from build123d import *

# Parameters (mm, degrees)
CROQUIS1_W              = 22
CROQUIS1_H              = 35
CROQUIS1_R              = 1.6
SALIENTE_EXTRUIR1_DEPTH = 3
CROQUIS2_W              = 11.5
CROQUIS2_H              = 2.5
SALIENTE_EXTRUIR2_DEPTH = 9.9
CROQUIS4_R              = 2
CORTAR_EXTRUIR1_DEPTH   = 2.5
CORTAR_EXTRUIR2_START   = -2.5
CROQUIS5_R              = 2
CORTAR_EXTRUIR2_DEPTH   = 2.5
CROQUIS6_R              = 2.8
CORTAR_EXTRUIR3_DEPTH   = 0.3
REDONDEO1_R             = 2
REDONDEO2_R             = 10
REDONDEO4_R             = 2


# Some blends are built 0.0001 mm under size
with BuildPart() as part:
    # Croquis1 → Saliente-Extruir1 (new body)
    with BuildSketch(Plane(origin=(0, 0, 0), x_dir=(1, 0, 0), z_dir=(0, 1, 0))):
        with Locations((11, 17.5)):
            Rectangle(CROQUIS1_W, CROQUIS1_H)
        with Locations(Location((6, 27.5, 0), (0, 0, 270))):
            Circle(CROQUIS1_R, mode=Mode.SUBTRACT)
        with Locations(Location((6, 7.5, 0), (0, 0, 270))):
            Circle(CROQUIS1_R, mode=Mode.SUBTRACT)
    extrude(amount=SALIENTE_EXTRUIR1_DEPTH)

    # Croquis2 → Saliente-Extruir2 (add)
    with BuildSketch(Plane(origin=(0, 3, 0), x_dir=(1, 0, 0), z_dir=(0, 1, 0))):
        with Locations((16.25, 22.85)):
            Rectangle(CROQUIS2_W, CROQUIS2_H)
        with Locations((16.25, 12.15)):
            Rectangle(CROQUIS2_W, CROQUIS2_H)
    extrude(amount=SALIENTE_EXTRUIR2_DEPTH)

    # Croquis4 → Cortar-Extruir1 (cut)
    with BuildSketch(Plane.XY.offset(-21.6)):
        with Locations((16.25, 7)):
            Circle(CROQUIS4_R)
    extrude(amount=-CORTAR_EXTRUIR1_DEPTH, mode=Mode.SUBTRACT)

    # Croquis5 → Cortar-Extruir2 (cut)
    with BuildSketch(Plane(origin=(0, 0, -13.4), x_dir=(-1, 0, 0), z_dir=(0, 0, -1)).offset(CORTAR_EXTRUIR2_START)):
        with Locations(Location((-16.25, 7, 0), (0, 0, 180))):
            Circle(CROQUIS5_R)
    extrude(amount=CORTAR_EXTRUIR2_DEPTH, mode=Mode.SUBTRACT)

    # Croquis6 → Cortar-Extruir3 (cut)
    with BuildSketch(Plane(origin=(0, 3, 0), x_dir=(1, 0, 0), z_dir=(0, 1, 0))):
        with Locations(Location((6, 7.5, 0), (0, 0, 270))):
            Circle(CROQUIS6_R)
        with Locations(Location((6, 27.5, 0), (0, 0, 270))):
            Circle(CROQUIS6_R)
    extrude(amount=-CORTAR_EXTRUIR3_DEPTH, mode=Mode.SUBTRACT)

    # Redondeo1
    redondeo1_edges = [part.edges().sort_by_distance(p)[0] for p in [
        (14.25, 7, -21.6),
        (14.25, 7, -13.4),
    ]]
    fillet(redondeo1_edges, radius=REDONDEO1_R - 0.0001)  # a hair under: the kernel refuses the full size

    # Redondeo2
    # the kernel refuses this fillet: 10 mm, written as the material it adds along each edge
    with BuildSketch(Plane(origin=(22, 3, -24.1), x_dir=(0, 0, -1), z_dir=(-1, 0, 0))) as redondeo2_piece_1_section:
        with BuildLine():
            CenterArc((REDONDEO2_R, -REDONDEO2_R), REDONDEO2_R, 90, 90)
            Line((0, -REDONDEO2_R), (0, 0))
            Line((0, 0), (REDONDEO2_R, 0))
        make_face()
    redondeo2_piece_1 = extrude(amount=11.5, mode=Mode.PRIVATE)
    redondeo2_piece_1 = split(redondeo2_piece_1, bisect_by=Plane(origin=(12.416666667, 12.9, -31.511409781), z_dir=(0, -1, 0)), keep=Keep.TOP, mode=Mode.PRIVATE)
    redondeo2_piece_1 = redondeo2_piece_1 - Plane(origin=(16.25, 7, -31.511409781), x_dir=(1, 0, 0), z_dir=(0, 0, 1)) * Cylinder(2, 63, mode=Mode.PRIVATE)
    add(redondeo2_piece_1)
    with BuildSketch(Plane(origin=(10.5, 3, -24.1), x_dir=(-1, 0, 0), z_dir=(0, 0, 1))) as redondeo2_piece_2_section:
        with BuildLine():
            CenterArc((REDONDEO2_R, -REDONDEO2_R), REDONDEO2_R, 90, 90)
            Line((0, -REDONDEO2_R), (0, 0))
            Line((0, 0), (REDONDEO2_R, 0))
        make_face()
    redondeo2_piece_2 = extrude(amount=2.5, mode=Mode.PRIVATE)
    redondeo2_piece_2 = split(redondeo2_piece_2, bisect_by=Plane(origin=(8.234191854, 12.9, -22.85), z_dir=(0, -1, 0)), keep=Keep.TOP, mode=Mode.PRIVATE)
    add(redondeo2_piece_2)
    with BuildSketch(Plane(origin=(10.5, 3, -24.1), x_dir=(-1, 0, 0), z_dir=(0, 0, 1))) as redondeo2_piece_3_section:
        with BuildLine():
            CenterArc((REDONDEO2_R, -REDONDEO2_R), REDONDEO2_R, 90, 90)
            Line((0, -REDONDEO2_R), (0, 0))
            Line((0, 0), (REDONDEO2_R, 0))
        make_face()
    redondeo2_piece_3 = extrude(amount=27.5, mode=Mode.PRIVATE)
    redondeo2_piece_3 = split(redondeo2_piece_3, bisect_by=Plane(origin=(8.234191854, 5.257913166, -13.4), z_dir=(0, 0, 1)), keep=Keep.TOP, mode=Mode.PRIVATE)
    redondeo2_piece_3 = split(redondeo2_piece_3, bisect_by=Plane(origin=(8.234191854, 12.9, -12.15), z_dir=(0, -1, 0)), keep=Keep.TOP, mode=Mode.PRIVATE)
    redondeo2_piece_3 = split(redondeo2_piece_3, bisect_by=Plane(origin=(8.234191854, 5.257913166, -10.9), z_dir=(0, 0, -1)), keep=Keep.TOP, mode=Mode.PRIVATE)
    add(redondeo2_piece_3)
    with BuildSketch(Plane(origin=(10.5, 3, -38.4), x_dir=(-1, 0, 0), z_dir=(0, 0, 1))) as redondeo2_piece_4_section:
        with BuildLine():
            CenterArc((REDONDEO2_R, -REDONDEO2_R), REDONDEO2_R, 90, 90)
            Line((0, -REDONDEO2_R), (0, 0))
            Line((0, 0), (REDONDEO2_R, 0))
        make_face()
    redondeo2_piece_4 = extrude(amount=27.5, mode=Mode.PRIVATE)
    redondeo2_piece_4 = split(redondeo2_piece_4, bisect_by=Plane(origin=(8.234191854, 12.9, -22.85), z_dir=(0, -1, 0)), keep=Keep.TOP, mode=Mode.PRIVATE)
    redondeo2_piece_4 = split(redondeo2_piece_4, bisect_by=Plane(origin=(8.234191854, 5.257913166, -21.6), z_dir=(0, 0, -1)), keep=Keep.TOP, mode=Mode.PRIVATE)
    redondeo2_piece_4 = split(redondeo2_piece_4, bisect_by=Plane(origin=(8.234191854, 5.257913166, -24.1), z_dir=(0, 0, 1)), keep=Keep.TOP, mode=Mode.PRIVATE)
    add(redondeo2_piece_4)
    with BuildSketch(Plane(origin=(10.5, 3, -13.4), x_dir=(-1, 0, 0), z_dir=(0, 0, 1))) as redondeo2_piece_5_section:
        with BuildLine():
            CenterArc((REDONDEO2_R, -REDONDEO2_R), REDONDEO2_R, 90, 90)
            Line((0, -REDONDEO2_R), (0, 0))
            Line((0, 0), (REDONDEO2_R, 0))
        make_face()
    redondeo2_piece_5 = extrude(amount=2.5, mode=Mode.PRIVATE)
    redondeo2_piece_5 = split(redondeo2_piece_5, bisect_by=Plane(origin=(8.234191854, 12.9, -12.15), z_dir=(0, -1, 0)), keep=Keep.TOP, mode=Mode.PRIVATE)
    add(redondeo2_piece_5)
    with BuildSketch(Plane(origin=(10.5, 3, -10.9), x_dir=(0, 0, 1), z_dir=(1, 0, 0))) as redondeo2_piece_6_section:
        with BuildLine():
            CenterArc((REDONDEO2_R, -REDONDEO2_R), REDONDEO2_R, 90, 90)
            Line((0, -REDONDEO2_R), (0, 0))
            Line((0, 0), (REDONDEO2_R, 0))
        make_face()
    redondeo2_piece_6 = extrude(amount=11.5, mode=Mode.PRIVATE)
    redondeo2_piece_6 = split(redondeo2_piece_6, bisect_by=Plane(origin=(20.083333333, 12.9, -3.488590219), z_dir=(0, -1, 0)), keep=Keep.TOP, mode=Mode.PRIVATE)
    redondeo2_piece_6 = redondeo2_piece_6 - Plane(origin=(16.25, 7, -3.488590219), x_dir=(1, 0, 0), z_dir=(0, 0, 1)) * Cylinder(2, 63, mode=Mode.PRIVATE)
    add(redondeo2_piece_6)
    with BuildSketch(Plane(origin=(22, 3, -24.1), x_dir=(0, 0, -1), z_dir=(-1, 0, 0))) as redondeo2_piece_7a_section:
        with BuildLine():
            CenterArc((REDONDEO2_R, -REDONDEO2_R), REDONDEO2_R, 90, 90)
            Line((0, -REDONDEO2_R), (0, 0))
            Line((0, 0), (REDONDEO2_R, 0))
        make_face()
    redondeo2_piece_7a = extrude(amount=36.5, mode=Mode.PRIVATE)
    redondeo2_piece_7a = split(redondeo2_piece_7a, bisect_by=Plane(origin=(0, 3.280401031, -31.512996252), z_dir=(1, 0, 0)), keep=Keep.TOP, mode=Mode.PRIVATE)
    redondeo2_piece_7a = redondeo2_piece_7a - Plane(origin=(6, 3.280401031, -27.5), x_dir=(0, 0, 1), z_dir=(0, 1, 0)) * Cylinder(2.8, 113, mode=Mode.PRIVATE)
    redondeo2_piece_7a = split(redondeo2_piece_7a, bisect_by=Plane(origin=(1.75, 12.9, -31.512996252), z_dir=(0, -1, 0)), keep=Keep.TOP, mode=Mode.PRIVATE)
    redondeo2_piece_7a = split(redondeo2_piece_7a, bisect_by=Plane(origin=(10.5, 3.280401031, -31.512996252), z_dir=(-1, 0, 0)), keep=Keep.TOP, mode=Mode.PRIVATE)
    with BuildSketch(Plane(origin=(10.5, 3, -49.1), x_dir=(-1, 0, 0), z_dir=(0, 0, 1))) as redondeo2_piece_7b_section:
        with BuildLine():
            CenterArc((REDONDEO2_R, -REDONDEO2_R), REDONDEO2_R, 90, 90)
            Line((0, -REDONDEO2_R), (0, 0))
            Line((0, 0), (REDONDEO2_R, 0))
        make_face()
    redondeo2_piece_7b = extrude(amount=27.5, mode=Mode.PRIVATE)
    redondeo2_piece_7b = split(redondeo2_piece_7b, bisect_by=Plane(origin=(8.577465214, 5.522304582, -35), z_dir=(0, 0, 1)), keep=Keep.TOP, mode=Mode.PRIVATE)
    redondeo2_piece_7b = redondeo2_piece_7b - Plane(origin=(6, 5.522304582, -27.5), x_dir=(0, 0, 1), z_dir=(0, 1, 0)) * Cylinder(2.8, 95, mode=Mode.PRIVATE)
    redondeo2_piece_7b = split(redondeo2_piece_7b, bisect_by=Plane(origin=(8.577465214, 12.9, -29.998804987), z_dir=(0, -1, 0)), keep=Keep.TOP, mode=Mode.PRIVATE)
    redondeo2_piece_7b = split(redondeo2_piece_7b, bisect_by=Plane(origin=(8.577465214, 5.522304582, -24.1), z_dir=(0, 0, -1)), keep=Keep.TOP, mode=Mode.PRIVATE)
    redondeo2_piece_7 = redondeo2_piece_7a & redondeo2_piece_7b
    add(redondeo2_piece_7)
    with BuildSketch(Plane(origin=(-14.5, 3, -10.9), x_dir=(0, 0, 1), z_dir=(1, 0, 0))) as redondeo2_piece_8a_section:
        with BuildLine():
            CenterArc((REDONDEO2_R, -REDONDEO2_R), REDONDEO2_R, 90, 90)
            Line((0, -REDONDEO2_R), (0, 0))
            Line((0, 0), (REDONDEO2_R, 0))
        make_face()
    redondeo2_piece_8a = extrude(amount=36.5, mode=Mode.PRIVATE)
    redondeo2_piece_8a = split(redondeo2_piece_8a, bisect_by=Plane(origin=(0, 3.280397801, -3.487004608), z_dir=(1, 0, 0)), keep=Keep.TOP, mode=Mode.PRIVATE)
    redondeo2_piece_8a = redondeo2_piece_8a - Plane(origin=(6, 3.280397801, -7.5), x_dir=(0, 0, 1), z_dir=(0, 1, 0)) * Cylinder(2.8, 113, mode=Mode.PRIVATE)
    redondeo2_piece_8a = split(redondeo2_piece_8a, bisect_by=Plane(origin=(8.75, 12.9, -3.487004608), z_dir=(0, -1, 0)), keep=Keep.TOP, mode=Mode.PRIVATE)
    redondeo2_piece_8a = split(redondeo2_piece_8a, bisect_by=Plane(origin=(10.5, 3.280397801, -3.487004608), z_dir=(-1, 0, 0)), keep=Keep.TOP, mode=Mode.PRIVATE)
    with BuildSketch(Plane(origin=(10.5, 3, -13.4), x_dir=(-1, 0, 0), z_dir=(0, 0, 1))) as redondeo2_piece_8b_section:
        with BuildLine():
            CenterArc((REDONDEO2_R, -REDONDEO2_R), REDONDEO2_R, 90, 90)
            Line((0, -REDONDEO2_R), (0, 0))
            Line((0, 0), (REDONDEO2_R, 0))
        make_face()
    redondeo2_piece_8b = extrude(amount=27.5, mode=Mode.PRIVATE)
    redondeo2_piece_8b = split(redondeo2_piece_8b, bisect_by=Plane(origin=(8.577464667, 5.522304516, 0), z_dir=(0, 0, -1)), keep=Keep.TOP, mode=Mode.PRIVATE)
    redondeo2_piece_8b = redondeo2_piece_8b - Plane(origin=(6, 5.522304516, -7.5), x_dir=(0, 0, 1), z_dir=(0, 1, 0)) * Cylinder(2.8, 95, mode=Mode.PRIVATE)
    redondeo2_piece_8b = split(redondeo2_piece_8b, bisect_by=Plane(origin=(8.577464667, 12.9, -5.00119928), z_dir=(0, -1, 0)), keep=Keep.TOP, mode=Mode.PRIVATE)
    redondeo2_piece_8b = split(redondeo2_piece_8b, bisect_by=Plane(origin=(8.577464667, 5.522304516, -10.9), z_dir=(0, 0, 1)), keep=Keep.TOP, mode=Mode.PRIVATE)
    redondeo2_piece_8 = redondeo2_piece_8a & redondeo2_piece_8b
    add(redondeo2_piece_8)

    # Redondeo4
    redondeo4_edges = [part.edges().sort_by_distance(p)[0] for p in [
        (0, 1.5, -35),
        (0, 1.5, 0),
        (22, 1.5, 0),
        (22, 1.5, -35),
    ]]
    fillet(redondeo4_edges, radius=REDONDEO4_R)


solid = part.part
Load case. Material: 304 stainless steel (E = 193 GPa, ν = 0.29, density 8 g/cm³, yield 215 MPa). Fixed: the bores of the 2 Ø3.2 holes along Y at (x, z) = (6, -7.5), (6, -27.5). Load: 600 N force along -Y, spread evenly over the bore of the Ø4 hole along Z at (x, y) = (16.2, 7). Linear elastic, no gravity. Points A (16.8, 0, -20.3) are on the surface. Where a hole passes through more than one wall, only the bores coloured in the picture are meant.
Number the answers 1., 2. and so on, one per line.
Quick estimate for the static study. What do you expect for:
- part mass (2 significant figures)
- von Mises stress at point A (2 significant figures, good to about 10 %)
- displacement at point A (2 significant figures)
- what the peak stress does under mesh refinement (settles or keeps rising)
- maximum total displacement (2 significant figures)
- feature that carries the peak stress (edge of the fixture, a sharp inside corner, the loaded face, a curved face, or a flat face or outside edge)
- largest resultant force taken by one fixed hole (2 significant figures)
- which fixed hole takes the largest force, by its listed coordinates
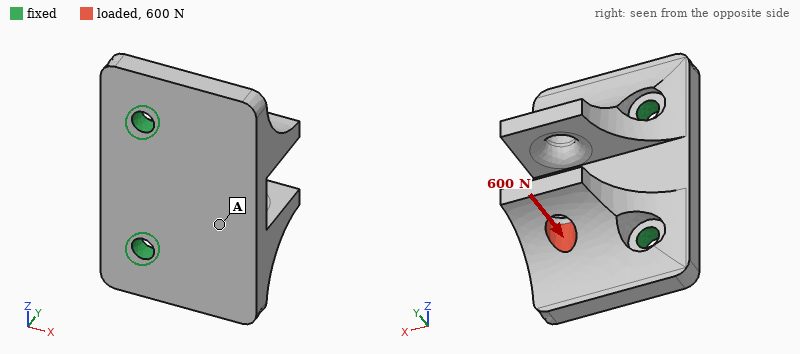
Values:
1. 27 g
2. 38 MPa
3. 17 µm
4. keeps rising
5. 32 µm
6. edge of the fixture
7. 510 N
8. (6, -27.5)
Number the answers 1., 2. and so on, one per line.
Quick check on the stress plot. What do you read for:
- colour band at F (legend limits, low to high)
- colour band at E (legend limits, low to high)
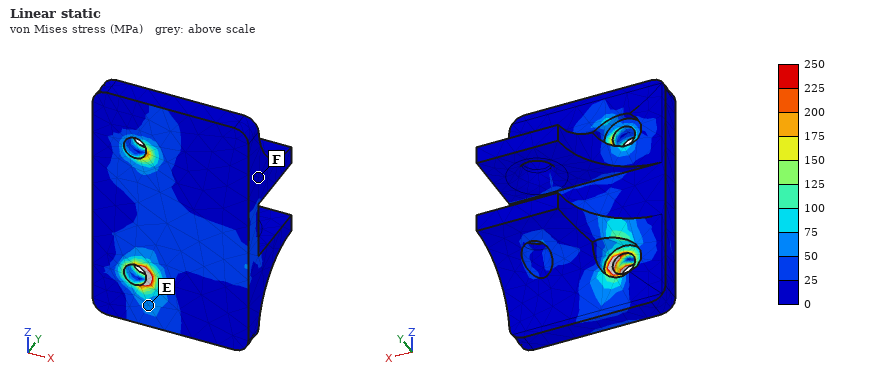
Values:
1. 0 to 25 MPa
2. 50 to 75 MPa
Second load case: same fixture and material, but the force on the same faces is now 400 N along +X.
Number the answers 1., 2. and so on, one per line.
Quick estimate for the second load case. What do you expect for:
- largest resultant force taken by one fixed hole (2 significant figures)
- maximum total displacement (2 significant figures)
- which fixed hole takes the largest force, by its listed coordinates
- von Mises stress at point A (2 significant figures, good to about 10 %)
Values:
1. 350 N
2. 12 µm
3. (6, -27.5)
4. 13 MPa
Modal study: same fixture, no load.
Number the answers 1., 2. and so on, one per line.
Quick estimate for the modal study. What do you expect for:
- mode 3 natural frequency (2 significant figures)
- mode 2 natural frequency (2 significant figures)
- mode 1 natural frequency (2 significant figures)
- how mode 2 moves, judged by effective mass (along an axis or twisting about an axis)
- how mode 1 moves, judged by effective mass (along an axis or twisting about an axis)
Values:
1. 17 kHz
2. 13 kHz
3. 7200 Hz
4. twisting about X
5. along Y
